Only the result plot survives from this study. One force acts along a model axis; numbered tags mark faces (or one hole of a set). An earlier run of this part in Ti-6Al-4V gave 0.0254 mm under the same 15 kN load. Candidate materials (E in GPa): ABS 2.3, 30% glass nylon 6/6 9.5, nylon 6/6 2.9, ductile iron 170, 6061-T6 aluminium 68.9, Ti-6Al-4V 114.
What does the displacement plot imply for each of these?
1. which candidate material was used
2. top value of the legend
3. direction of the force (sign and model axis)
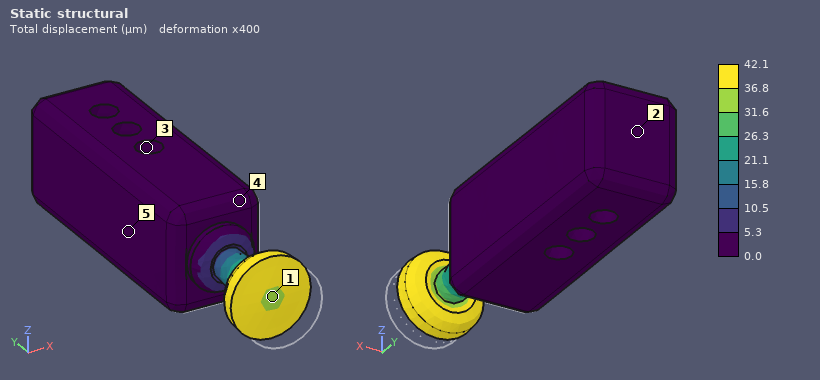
6061-T6 aluminium
42.1 µm
+Y
